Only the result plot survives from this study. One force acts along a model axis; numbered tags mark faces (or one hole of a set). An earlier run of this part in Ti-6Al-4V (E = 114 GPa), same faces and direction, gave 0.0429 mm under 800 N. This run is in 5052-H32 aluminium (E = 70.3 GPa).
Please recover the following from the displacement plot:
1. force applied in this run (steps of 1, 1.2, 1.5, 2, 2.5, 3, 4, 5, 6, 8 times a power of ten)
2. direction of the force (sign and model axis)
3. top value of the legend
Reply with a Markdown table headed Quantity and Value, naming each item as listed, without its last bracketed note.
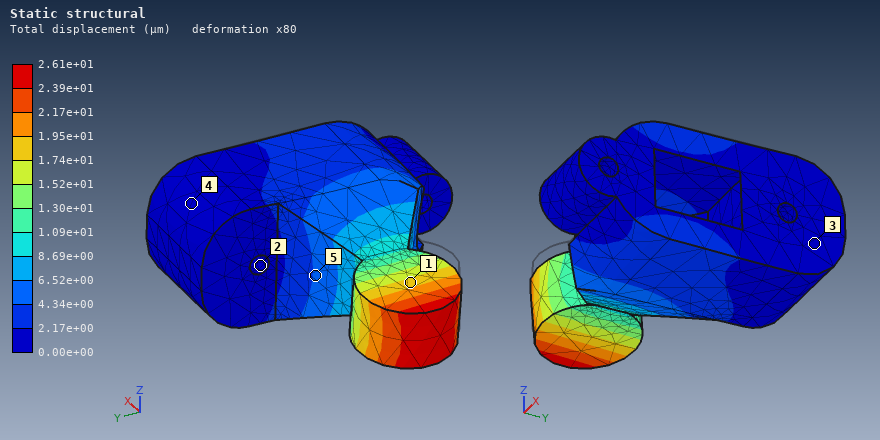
| Quantity | Value |
|---|---|
| force applied in this run | 300 N |
| direction of the force | -Z |
| top value of the legend | 2.61e+01 µm |
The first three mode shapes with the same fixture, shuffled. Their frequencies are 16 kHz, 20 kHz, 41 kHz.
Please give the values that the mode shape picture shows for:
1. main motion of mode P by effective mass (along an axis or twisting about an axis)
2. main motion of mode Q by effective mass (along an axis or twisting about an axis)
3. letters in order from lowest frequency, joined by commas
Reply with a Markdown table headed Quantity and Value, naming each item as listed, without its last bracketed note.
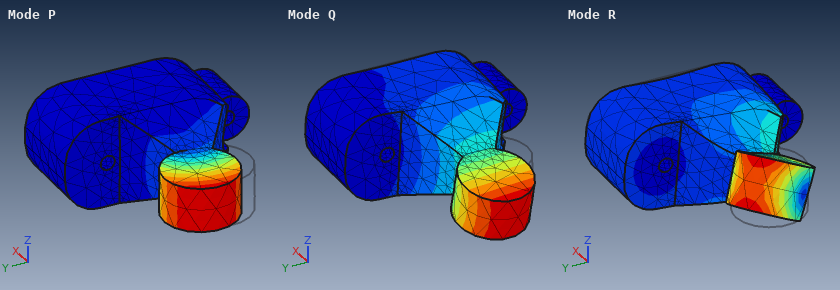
| Quantity | Value |
|---|---|
| main motion of mode P by effective mass | along Y |
| main motion of mode Q by effective mass | along Z |
| letters in order from lowest frequency, joined by commas | Q, P, R |
